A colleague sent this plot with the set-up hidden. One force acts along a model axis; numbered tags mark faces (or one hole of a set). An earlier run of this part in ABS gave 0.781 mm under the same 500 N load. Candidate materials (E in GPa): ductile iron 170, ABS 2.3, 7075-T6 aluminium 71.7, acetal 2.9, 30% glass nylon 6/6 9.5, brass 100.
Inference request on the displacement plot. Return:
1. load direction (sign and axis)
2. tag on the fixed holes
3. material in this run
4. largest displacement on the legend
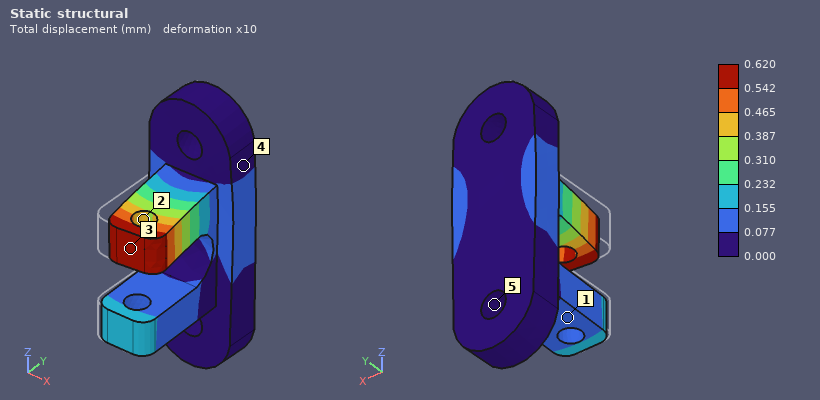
+X
5
acetal
0.620 mm
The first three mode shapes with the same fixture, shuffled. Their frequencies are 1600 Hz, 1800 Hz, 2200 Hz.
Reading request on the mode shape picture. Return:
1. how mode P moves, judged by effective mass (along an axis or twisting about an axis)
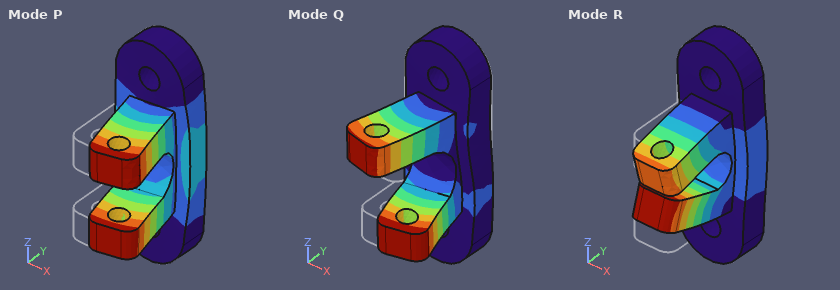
along X
